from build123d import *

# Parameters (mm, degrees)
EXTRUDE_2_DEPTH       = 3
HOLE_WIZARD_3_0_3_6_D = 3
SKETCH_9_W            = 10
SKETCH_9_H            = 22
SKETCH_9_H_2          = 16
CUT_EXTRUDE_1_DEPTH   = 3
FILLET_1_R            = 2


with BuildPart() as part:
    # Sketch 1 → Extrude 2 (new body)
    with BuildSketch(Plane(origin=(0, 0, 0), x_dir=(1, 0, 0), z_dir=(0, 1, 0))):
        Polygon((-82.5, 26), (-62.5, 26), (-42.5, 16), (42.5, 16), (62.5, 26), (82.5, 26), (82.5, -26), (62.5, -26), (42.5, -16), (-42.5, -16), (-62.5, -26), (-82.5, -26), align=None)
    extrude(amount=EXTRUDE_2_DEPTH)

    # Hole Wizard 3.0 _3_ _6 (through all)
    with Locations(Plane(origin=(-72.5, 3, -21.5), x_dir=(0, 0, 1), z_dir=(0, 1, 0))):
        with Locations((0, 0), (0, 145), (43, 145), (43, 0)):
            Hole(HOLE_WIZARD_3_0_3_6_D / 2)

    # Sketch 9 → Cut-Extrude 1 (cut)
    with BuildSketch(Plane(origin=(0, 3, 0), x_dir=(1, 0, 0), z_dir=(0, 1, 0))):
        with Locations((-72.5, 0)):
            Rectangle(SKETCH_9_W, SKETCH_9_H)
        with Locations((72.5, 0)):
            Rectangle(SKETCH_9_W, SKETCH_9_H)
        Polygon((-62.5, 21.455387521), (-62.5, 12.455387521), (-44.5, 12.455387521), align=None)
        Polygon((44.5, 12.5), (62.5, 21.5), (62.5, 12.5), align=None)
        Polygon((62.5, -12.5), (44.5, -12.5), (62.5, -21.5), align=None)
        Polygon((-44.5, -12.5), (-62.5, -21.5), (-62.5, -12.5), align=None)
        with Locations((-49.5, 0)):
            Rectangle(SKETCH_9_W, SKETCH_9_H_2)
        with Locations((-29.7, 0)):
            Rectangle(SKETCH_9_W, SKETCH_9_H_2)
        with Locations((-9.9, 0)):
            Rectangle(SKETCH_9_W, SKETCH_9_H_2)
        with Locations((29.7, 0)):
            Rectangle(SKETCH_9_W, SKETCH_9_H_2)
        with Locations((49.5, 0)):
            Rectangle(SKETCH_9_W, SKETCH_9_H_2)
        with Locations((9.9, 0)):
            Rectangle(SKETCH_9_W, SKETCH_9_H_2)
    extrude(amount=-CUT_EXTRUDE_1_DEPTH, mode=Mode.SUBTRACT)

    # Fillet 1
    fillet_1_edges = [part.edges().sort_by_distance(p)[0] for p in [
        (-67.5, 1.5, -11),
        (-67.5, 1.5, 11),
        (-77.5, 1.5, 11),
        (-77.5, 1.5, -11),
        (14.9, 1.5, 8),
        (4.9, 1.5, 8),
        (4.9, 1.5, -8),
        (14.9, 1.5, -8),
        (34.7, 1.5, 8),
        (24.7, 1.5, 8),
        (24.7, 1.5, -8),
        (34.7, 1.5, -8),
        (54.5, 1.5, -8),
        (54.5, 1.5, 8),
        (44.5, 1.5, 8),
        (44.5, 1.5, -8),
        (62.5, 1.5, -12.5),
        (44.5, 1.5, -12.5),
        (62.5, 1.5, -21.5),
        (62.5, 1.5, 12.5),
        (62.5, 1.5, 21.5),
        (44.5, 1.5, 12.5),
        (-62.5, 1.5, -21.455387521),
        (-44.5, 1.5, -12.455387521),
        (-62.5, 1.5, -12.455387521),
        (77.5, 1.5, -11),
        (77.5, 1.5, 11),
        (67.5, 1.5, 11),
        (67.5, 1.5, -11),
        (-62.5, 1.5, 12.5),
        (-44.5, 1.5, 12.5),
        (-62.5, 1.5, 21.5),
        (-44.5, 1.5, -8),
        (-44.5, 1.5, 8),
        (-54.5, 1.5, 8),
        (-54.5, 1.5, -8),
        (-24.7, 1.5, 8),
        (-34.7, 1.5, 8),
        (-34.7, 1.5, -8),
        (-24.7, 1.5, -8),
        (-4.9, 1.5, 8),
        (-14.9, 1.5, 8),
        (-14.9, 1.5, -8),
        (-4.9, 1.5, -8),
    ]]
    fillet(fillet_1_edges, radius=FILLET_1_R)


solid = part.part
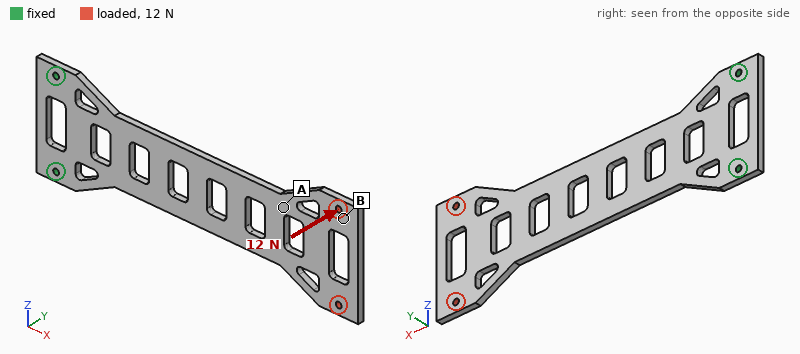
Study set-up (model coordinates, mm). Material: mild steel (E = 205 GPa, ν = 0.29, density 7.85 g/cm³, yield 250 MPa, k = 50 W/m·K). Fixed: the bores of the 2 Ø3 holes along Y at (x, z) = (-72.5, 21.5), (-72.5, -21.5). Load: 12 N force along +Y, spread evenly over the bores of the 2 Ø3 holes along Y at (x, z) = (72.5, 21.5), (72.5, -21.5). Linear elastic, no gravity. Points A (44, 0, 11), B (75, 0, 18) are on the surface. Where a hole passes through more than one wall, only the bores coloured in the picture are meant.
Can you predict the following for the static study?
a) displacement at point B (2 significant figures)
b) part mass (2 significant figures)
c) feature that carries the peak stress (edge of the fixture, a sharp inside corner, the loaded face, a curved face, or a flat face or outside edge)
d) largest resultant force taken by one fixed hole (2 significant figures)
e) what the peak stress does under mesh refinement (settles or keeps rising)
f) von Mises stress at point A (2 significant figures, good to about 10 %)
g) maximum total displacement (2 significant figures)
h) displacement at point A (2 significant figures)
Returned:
1.4 mm
110 g
edge of the fixture
6.0 N
keeps rising
12 MPa
1.5 mm
0.94 mm
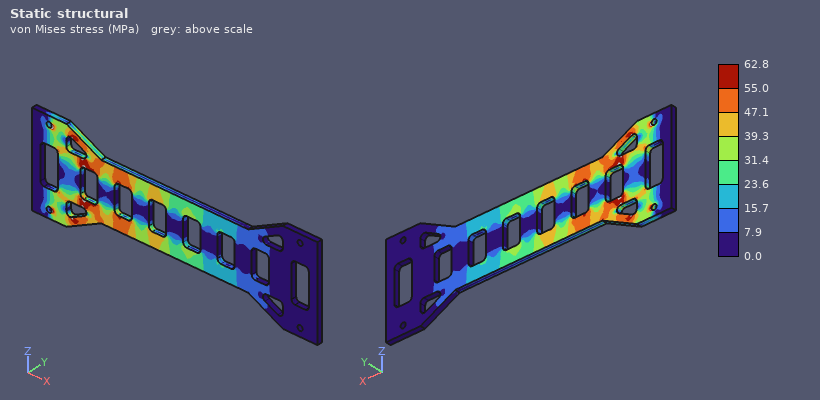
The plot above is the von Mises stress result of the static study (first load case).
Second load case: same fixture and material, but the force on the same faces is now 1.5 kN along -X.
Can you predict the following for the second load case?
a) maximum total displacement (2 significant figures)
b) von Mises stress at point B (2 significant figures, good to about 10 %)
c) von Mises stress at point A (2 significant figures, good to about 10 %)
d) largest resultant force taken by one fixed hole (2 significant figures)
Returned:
22 µm
18 MPa
22 MPa
780 N
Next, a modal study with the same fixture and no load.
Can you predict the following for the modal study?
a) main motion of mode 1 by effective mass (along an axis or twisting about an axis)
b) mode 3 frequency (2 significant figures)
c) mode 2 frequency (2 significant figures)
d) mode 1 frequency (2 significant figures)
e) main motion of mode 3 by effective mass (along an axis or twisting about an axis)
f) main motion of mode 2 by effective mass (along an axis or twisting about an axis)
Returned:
along Y
590 Hz
540 Hz
81 Hz
twisting about X
along Y
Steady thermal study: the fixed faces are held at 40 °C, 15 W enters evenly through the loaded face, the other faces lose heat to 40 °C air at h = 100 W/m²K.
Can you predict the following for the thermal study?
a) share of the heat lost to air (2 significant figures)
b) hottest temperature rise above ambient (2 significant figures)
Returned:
100 %
65 K
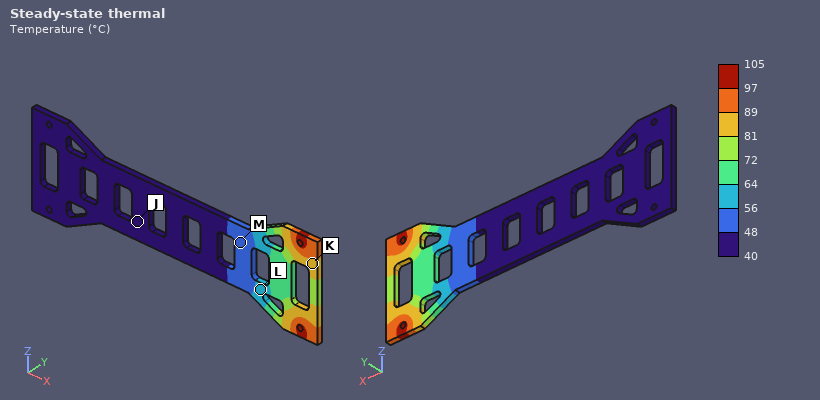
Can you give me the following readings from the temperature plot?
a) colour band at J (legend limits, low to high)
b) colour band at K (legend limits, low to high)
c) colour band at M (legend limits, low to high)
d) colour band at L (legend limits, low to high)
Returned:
40 to 48 °C
81 to 89 °C
48 to 56 °C
56 to 64 °C
